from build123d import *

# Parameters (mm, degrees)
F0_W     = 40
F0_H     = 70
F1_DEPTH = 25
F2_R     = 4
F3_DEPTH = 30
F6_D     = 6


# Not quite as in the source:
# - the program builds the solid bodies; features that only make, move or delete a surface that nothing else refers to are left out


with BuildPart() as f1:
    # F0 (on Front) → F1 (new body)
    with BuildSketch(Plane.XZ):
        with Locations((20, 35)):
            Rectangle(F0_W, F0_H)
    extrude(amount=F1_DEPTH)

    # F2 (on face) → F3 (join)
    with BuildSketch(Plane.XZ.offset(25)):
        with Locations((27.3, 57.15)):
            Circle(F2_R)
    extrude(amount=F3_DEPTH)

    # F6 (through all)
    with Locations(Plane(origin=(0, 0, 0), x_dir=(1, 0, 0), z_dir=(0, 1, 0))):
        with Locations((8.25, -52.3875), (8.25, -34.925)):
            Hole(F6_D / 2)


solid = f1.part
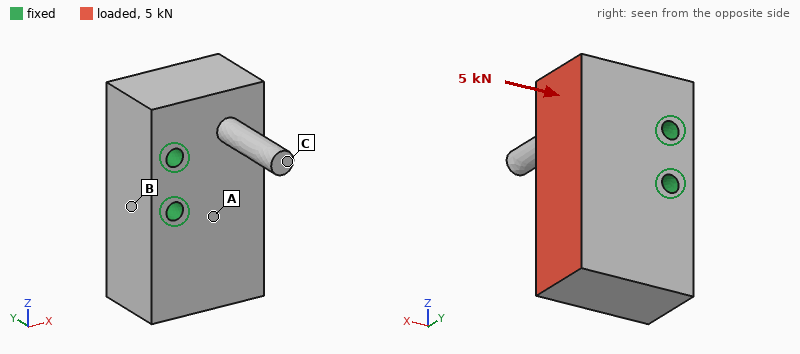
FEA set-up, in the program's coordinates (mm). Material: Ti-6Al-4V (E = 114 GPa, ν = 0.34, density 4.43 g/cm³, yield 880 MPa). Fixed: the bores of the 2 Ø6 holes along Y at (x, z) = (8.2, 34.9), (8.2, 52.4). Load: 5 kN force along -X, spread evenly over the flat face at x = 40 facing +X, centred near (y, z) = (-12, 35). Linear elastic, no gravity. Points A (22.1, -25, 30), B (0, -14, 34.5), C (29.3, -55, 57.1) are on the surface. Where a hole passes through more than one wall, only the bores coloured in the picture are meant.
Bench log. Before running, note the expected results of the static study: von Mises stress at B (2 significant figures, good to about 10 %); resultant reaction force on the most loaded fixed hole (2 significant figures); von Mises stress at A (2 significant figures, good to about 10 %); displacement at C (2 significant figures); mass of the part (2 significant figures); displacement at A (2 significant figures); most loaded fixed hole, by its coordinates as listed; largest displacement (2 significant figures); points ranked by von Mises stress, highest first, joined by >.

9.9 MPa
4.3 kN
6.1 MPa
1.0 µm
310 g
1.7 µm
(8.2, 34.9)
6.3 µm
B > A > C
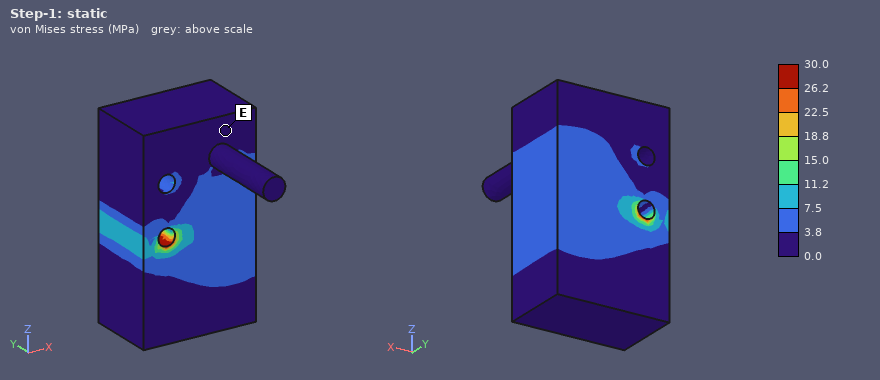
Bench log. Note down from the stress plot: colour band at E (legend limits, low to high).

0.0 to 3.8 MPa
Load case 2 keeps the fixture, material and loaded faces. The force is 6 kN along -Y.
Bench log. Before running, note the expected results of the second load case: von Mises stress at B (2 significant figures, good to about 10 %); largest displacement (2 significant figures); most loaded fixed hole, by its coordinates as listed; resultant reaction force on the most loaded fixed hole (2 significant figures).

10 MPa
23 µm
(8.2, 34.9)
3.9 kN
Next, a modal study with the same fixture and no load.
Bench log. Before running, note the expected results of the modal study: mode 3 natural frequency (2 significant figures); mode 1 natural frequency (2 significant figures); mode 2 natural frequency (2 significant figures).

8300 Hz
5400 Hz
5400 Hz
